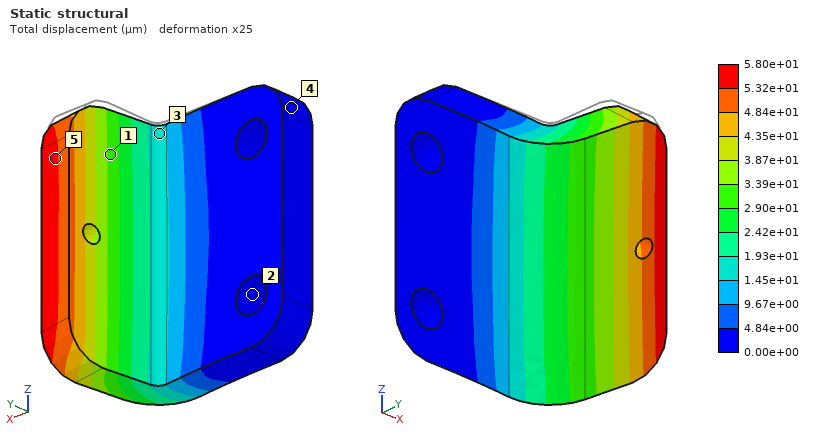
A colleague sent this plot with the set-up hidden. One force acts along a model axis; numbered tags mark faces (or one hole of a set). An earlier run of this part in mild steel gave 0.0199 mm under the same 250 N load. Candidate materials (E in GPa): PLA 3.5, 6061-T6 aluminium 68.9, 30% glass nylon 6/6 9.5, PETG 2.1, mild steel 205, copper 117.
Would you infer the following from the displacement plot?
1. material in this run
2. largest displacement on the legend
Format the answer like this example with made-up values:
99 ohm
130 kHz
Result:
6061-T6 aluminium
5.80e+01 µm
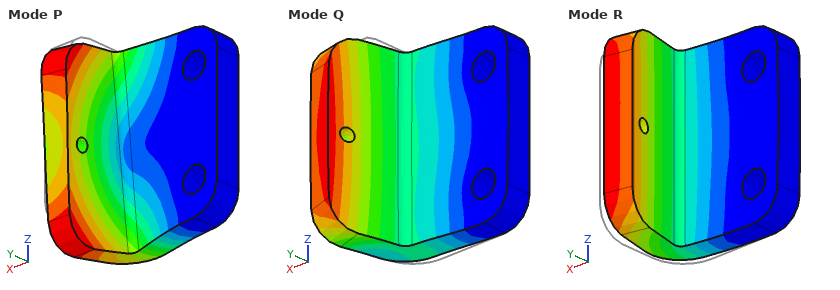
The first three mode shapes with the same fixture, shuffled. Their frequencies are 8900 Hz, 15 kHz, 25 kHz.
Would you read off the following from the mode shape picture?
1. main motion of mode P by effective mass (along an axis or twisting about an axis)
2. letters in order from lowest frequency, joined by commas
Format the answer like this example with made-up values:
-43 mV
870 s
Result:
along Z
R, P, Q
